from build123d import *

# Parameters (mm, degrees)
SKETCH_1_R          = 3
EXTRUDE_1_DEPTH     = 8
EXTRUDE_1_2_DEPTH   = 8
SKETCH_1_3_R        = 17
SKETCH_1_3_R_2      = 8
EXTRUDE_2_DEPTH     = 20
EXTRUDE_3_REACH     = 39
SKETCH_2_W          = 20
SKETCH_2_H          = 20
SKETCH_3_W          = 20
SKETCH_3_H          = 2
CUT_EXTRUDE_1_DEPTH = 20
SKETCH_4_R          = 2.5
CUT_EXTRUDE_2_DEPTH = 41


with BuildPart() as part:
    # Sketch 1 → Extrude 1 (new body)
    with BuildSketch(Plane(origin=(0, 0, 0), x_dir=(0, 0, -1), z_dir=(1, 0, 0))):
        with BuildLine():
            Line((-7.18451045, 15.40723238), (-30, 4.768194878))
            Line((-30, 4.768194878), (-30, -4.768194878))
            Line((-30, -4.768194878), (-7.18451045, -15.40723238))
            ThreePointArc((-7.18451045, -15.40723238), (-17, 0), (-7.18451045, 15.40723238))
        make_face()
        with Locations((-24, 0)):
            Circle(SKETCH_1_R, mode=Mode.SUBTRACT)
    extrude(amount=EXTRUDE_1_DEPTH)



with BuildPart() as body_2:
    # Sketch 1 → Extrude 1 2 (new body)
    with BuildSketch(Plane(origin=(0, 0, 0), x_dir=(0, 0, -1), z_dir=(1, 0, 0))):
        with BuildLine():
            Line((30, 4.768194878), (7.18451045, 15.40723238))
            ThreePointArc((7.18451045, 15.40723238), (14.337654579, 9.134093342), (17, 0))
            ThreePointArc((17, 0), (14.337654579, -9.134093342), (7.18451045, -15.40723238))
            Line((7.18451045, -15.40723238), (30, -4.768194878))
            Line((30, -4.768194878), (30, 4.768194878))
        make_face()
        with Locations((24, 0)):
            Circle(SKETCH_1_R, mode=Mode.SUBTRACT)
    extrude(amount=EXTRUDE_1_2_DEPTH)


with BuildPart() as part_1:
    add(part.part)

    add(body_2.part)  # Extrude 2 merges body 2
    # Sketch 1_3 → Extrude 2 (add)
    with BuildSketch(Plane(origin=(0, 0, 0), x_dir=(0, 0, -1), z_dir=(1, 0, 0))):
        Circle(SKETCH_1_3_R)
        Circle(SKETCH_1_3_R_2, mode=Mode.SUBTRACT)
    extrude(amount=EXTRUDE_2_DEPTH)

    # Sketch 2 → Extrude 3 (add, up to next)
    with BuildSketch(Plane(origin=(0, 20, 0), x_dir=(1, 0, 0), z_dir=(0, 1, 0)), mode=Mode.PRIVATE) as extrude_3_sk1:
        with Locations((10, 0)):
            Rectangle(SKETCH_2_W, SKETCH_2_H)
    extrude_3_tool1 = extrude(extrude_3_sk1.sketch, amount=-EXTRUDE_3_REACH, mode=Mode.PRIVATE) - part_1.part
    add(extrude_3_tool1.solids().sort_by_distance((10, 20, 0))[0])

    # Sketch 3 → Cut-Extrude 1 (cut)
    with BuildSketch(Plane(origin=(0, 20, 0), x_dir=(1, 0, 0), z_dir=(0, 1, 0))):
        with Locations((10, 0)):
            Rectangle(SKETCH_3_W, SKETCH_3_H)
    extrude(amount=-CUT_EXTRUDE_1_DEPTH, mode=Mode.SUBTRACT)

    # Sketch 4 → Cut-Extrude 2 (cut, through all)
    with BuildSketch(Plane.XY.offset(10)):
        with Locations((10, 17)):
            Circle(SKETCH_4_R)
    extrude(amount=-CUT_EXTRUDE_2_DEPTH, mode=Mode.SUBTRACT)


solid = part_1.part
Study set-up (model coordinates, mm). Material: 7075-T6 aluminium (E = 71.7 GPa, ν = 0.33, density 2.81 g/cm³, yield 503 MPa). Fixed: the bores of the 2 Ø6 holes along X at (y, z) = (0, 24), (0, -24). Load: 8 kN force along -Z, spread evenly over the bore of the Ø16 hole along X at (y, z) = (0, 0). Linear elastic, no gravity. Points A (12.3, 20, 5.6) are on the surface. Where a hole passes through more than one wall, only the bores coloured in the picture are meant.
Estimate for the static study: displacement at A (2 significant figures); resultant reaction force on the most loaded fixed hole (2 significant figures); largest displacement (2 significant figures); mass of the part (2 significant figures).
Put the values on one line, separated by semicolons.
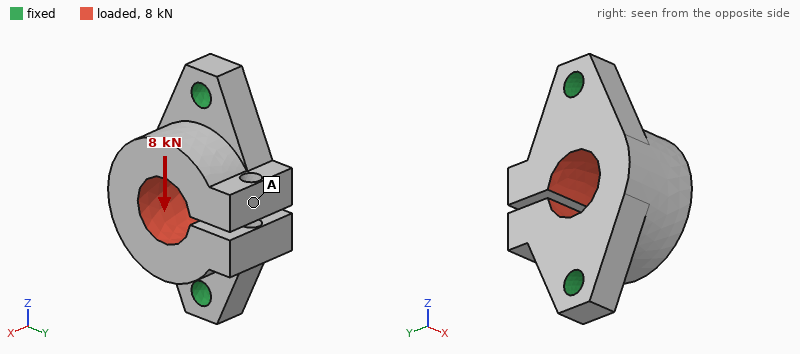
32 µm; 4.1 kN; 46 µm; 52 g
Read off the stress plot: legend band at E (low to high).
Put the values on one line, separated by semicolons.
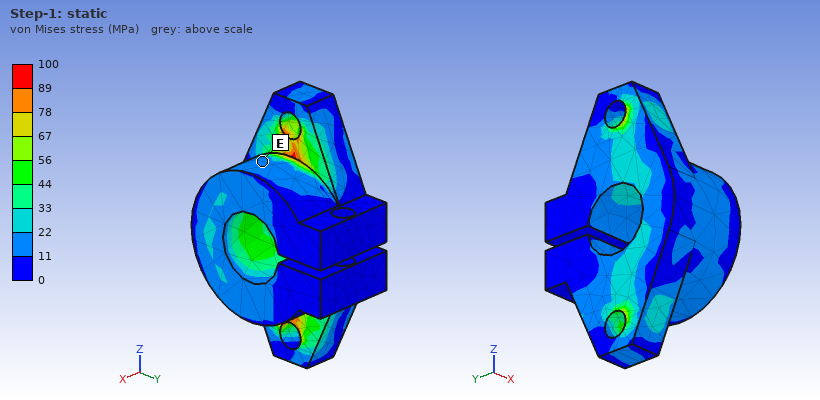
11 to 22 MPa
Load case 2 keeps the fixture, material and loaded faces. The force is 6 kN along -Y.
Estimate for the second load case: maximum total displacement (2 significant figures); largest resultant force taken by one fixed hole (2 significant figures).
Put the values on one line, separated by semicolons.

87 µm; 3.9 kN
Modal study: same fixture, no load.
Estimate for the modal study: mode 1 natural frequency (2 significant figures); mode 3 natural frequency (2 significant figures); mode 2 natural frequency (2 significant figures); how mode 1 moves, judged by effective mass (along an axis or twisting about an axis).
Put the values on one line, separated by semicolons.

7000 Hz; 8900 Hz; 8400 Hz; along Y
